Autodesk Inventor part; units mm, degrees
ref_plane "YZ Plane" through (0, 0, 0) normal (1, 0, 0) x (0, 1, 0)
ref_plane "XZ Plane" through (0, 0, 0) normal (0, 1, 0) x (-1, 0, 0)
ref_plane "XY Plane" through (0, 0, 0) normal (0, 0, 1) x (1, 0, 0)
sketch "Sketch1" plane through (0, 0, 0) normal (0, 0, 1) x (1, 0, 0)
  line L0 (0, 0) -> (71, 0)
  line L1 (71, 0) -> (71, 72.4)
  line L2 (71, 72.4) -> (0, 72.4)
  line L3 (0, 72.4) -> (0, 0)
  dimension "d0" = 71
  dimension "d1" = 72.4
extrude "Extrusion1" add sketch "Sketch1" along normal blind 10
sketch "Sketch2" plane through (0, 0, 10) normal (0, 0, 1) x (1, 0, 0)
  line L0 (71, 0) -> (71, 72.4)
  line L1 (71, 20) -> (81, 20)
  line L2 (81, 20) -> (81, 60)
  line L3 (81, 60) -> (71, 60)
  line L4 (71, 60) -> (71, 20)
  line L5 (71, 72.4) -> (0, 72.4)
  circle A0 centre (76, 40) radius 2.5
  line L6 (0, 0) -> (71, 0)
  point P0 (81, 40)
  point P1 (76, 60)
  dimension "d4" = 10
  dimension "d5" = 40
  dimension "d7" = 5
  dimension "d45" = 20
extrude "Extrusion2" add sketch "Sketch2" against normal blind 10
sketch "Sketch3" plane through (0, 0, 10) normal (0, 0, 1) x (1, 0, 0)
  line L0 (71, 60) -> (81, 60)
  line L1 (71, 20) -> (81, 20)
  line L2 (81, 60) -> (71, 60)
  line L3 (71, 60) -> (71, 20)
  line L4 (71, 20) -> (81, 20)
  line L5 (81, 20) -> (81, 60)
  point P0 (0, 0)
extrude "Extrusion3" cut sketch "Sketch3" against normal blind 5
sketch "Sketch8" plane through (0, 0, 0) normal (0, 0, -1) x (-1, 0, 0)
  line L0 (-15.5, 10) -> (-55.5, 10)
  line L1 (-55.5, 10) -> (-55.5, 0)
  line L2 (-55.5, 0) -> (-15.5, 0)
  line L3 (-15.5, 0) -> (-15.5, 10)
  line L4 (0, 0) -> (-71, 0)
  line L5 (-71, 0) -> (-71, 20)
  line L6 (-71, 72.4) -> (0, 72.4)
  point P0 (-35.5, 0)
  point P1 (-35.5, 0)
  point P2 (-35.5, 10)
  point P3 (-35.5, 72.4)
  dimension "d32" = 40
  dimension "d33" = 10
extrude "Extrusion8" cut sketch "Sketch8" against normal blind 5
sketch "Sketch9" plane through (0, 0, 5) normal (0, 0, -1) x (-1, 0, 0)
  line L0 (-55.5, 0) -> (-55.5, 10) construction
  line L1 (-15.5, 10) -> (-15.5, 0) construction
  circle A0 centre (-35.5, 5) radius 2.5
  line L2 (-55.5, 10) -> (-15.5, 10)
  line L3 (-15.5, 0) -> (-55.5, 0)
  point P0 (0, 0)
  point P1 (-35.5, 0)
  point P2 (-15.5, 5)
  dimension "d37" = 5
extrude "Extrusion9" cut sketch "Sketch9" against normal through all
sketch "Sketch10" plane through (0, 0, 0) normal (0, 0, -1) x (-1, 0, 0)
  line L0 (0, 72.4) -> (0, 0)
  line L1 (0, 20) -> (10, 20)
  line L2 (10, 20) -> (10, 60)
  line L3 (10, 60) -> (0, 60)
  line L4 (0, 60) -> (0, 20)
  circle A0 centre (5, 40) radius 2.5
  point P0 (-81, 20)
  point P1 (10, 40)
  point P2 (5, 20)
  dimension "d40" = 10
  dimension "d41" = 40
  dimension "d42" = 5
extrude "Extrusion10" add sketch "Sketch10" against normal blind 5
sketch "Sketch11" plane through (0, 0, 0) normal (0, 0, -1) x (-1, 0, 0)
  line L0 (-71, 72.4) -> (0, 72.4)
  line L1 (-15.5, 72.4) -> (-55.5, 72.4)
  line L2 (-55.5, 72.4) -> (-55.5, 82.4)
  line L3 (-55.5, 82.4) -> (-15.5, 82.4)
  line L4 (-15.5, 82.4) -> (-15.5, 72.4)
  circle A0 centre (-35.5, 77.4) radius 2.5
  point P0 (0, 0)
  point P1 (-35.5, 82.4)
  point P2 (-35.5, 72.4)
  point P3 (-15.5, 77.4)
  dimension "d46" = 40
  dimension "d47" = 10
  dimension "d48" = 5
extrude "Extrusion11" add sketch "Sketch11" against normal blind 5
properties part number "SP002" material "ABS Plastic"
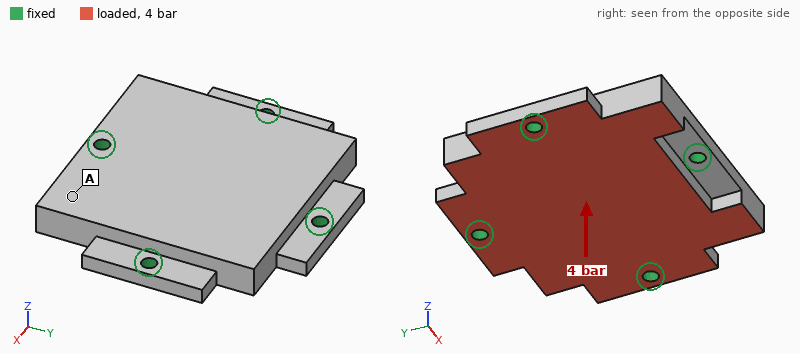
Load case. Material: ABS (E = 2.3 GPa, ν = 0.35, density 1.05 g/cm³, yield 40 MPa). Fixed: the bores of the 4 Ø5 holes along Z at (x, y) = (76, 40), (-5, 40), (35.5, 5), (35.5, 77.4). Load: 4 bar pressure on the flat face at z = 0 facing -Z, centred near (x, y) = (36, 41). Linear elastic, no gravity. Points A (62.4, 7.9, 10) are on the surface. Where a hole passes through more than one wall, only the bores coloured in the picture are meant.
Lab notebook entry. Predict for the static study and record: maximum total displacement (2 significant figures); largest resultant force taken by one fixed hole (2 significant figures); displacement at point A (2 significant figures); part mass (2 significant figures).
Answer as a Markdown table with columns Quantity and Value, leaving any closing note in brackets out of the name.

| Quantity | Value |
|---|---|
| maximum total displacement | 0.27 mm |
| largest resultant force taken by one fixed hole | 670 N |
| displacement at point A | 0.22 mm |
| part mass | 58 g |
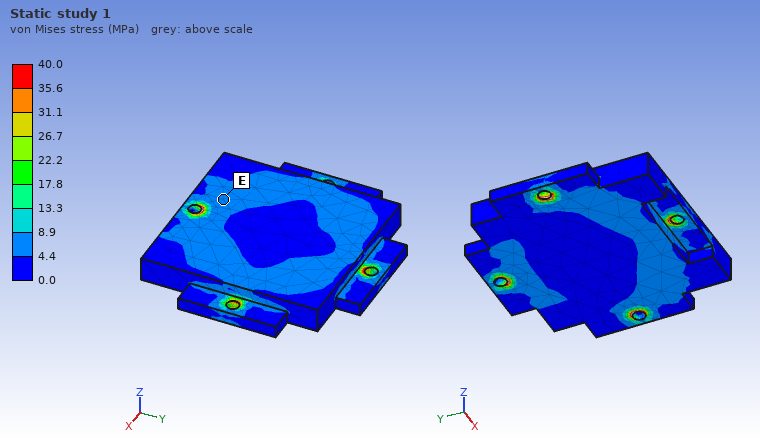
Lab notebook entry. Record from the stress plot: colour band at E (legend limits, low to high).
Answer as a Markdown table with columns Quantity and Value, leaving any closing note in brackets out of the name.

| Quantity | Value |
|---|---|
| colour band at E | 4.4 to 8.9 MPa |
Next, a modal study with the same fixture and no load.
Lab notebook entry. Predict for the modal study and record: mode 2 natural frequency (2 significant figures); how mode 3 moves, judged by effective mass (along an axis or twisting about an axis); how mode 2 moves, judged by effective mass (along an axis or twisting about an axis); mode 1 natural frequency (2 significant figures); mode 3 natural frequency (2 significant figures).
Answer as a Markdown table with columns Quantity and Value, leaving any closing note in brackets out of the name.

| Quantity | Value |
|---|---|
| mode 2 natural frequency | 2200 Hz |
| how mode 3 moves, judged by effective mass | along Z |
| how mode 2 moves, judged by effective mass | along Z |
| mode 1 natural frequency | 2000 Hz |
| mode 3 natural frequency | 2400 Hz |
